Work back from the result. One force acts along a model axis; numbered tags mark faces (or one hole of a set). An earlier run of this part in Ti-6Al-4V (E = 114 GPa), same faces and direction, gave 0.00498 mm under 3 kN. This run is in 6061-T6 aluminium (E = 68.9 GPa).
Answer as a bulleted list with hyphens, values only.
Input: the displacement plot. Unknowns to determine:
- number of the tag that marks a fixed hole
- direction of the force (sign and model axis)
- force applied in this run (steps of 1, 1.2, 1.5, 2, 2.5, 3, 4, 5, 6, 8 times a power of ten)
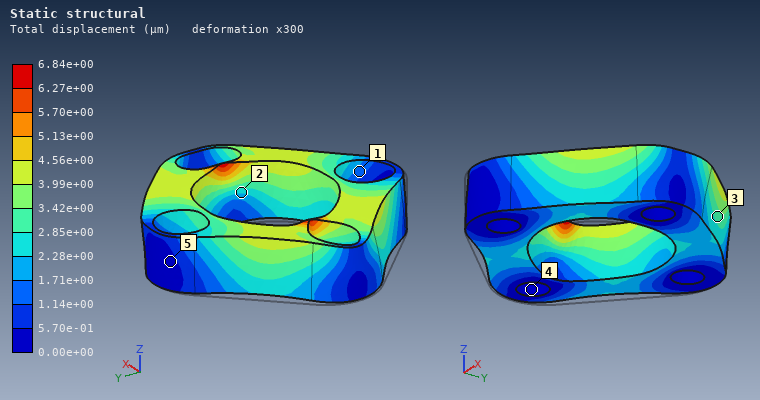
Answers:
- 4
- +X
- 2.5 kN
